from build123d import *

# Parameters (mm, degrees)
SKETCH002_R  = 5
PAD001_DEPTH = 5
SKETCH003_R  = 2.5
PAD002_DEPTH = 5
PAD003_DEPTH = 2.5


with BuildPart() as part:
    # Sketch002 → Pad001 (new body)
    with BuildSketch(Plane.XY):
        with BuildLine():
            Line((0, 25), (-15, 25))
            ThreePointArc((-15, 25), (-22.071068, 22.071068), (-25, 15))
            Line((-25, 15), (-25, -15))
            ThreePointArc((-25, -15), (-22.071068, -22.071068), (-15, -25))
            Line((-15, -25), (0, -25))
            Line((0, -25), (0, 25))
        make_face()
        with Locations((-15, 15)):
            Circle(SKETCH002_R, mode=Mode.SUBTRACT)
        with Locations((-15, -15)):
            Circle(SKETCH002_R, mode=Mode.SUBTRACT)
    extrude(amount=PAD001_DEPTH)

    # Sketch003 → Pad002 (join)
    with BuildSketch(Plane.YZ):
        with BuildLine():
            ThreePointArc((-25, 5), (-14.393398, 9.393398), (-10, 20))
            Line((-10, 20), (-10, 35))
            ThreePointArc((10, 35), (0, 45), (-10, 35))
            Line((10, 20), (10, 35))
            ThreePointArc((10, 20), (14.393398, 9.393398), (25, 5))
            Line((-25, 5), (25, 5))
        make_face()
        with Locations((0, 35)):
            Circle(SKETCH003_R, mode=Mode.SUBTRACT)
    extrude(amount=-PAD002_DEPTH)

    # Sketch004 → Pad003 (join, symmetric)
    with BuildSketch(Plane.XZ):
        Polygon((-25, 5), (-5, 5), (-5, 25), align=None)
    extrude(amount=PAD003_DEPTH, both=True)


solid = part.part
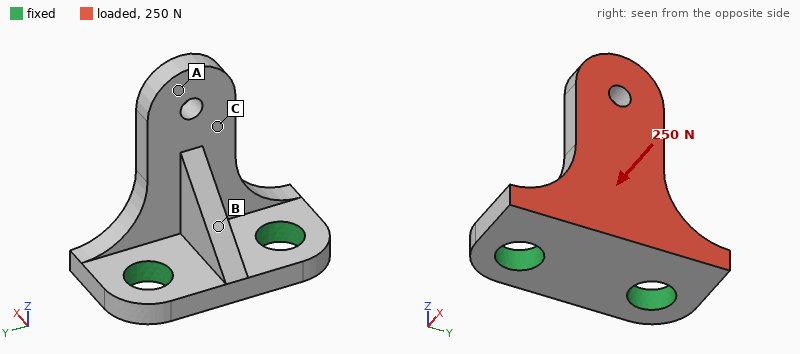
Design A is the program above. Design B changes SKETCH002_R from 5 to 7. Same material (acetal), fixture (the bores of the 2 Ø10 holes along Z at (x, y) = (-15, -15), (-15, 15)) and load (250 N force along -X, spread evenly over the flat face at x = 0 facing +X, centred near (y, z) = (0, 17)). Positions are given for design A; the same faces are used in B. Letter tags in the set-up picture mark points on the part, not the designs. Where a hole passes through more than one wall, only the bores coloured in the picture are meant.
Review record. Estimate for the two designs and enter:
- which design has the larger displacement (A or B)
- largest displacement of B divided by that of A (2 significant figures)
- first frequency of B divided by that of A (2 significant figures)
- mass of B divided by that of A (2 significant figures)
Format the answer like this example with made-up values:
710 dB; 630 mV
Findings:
A; 0.83; 1.1; 0.93
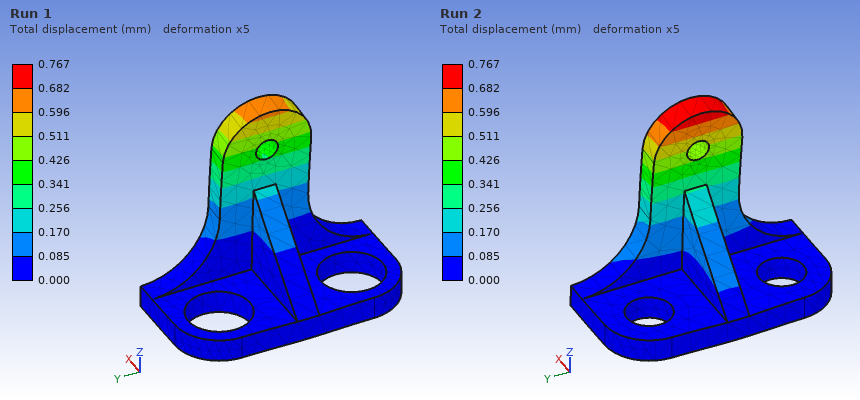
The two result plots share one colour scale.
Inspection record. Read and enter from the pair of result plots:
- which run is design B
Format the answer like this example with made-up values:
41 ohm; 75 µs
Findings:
Run 1
